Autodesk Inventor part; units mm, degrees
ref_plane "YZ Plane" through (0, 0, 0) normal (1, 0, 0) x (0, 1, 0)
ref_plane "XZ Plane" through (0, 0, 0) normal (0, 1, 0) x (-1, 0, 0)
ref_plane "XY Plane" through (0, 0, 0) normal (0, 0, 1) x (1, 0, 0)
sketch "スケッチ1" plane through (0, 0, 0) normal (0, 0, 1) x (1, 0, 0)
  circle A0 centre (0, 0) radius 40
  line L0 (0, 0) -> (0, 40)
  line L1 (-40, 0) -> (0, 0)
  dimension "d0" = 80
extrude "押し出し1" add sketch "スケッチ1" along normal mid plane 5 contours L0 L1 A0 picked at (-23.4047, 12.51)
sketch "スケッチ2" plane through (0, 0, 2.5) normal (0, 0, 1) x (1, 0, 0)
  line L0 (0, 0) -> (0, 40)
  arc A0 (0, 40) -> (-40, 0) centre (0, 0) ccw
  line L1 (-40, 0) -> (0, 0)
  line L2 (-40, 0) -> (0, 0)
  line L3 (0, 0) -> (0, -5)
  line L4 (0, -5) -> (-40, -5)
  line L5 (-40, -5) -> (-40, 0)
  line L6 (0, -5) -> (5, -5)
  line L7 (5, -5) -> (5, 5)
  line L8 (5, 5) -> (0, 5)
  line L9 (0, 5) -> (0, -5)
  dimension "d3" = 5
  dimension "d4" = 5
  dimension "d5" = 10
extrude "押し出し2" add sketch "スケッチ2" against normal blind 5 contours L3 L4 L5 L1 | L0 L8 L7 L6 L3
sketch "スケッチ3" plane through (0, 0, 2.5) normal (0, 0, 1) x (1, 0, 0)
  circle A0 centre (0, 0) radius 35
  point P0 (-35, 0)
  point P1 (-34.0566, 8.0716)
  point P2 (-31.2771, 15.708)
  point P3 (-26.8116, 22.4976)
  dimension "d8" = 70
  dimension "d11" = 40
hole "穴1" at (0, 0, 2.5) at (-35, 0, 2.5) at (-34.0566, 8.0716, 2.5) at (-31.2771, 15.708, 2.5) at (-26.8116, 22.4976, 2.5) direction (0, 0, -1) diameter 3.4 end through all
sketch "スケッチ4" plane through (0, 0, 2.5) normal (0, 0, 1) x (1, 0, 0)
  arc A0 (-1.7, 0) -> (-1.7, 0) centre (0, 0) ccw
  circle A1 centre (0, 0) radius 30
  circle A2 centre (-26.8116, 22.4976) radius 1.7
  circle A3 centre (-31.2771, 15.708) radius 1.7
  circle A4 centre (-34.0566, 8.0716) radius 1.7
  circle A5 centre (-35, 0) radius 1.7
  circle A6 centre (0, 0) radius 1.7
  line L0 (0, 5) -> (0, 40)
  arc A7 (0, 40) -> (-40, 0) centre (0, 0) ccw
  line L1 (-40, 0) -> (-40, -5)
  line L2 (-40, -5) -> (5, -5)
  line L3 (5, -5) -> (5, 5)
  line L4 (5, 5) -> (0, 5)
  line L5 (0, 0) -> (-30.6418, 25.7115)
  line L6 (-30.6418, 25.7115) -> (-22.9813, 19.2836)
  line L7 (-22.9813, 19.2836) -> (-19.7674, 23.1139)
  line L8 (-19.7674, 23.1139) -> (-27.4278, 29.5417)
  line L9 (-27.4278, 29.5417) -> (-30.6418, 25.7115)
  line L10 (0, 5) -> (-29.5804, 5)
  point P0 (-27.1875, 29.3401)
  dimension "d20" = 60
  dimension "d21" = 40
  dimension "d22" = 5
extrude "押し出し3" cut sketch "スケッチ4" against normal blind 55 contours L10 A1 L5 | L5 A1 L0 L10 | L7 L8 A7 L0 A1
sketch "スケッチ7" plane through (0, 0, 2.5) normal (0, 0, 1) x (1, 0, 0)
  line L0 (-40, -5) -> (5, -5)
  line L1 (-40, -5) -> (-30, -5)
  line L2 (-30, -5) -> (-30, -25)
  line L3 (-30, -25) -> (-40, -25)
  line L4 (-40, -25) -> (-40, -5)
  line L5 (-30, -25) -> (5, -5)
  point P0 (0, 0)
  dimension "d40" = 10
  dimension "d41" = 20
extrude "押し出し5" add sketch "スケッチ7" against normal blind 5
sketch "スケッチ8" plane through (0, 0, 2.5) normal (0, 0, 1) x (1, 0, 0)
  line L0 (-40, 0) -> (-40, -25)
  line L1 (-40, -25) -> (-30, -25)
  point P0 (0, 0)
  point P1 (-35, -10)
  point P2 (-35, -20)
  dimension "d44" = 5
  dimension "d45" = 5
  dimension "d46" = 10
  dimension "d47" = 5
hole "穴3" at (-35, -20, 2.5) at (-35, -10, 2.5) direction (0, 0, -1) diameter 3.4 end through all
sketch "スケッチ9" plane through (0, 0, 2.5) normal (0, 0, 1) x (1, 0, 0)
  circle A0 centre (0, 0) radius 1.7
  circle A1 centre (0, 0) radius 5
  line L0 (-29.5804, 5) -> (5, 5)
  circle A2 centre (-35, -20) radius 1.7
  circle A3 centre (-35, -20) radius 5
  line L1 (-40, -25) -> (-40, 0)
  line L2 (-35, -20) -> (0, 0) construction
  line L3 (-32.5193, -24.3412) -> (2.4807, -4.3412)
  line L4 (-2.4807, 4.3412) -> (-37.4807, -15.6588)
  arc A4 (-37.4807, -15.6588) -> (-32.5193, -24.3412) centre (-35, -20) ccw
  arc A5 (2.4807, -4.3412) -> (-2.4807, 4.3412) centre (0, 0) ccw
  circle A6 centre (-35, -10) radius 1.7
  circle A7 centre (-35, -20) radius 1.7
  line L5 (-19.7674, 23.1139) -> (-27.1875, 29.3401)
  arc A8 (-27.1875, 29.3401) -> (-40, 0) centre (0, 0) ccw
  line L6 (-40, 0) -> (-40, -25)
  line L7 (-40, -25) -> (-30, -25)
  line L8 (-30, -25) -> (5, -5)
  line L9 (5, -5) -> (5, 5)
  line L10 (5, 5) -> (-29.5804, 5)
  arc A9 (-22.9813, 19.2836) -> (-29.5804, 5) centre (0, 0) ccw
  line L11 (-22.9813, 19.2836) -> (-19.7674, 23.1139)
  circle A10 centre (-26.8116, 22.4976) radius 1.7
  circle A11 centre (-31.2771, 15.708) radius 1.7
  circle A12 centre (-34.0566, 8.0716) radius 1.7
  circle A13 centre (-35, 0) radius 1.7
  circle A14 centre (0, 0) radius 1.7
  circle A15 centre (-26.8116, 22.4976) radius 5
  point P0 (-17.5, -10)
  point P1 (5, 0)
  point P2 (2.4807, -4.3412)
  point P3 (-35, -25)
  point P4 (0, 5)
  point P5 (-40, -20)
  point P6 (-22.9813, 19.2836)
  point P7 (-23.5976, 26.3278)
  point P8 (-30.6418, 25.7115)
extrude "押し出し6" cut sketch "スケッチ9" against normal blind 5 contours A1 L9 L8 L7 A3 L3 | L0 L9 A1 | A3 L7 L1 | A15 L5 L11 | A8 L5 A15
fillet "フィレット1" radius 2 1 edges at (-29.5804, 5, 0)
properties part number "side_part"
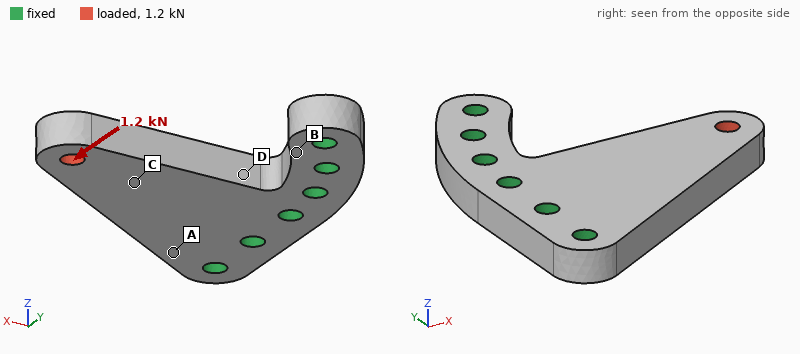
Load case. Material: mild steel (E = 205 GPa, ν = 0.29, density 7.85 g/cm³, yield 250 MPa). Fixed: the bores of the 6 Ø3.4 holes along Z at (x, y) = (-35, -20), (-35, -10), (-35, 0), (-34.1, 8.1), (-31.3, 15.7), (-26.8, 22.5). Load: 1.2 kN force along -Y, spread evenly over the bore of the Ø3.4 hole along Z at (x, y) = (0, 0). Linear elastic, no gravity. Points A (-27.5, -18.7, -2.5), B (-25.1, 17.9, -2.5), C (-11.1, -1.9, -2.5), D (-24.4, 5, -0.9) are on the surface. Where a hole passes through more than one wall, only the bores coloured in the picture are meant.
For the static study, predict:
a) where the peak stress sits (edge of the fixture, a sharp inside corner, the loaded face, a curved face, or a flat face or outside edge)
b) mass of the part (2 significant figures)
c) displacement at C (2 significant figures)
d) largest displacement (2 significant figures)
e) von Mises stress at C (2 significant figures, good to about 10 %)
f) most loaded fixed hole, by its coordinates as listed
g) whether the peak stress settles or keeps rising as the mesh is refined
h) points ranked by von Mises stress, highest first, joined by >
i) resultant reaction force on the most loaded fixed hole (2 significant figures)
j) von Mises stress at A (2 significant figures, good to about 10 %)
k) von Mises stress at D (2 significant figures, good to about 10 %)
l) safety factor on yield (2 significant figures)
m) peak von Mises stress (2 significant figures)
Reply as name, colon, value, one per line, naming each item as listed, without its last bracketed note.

where the peak stress sits: a curved face
mass of the part: 42 g
displacement at C: 9.0 µm
largest displacement: 26 µm
von Mises stress at C: 24 MPa
most loaded fixed hole, by its coordinates as listed: (-35, -20)
whether the peak stress settles or keeps rising as the mesh is refined: settles
points ranked by von Mises stress, highest first, joined by >: D > A > C > B
resultant reaction force on the most loaded fixed hole: 1.6 kN
von Mises stress at A: 44 MPa
von Mises stress at D: 71 MPa
safety factor on yield: 1.8
peak von Mises stress: 140 MPa
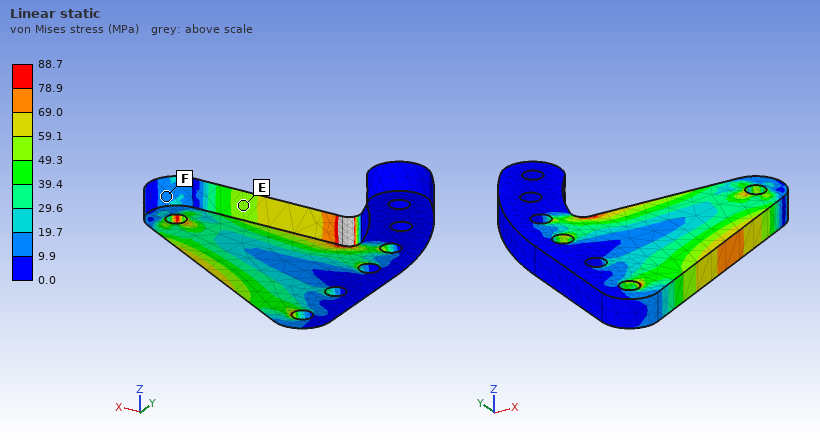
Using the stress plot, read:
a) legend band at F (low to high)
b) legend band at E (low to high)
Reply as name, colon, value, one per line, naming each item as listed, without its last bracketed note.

legend band at F: 9.9 to 19.7 MPa
legend band at E: 49.3 to 59.1 MPa
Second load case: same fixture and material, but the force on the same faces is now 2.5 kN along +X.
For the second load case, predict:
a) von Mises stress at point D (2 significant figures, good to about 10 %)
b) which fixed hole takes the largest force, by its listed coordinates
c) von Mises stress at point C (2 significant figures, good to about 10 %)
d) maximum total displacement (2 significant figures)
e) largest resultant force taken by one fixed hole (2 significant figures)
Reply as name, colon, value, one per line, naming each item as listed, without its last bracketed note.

von Mises stress at point D: 62 MPa
which fixed hole takes the largest force, by its listed coordinates: (-35, 0)
von Mises stress at point C: 38 MPa
maximum total displacement: 14 µm
largest resultant force taken by one fixed hole: 1.4 kN
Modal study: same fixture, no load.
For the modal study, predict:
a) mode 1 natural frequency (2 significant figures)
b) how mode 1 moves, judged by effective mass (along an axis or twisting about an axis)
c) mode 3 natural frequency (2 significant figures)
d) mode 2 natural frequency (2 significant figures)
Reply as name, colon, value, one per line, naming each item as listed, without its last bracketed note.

mode 1 natural frequency: 3900 Hz
how mode 1 moves, judged by effective mass: along Z
mode 3 natural frequency: 16 kHz
mode 2 natural frequency: 16 kHz
